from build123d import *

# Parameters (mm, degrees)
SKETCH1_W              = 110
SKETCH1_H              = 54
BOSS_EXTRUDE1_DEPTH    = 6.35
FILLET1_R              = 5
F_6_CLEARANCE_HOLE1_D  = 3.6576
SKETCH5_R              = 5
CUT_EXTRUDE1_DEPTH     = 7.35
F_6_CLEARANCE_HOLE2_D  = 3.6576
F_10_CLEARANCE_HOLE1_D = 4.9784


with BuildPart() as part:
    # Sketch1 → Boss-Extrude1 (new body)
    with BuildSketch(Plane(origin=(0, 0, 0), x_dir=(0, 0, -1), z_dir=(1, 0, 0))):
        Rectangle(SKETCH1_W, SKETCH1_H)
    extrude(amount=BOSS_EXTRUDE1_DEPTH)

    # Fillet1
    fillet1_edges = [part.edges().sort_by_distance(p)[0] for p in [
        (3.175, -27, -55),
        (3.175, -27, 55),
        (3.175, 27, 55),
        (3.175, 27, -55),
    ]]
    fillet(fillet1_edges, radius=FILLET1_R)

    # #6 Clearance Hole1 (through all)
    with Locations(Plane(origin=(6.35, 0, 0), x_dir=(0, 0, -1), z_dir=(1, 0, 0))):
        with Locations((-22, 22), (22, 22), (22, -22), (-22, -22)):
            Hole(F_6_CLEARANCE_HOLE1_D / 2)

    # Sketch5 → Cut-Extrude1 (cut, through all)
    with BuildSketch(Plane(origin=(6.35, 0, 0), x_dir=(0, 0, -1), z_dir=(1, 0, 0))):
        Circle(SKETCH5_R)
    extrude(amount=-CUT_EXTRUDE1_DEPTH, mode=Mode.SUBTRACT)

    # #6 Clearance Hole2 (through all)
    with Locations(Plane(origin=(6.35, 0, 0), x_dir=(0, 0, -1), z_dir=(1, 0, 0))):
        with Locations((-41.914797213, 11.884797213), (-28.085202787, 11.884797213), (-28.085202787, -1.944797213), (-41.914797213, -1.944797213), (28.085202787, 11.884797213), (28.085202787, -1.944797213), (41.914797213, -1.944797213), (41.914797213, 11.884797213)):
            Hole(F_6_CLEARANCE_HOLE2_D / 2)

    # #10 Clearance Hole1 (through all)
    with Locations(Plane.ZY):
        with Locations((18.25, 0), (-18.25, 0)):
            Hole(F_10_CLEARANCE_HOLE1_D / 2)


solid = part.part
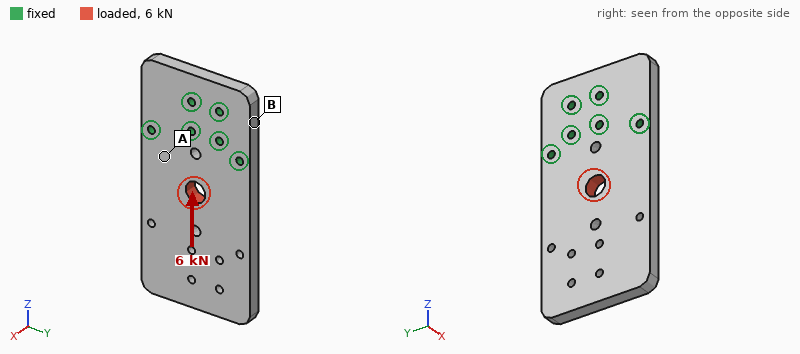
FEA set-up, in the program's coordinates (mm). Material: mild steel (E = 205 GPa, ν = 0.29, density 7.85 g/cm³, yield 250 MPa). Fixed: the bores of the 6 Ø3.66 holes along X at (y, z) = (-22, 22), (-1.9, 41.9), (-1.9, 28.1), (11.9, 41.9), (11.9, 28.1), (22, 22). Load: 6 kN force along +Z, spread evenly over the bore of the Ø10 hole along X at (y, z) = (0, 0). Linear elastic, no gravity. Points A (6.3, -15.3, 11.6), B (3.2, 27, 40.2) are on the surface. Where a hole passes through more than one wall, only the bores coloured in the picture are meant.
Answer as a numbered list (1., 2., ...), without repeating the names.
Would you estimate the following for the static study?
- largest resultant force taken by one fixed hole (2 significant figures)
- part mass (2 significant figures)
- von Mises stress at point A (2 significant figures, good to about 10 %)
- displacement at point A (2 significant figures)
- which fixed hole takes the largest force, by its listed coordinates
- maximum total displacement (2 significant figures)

1. 1.9 kN
2. 280 g
3. 18 MPa
4. 1.3 µm
5. (-22, 22)
6. 4.2 µm
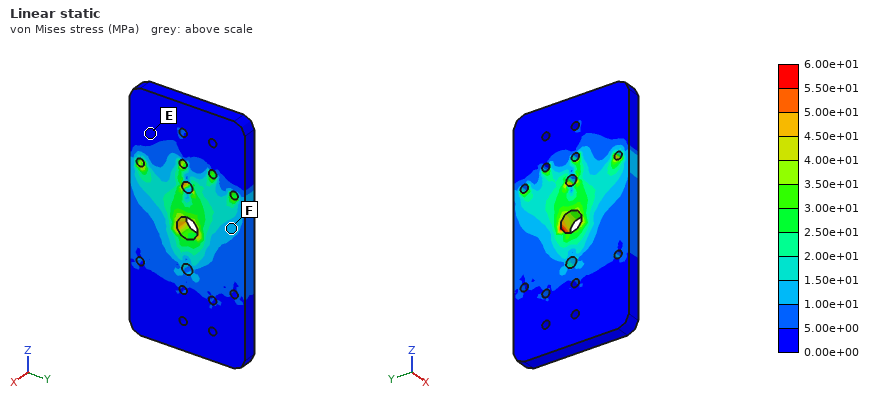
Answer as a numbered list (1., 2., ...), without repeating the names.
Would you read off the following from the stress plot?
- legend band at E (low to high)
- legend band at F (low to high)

1. 0.00e+00 to 5.00e+00 MPa
2. 1.00e+01 to 1.50e+01 MPa
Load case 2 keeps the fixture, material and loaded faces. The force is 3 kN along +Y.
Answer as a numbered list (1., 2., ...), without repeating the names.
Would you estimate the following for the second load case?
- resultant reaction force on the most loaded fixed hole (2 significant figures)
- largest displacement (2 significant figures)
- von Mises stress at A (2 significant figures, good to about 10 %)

1. 1.9 kN
2. 6.7 µm
3. 19 MPa
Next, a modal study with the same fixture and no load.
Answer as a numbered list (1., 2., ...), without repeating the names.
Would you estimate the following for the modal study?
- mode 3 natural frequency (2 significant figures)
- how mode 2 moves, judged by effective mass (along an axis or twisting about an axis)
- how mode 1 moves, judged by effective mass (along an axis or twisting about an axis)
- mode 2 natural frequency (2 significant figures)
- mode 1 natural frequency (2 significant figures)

1. 5000 Hz
2. twisting about Z
3. along X
4. 2700 Hz
5. 820 Hz
